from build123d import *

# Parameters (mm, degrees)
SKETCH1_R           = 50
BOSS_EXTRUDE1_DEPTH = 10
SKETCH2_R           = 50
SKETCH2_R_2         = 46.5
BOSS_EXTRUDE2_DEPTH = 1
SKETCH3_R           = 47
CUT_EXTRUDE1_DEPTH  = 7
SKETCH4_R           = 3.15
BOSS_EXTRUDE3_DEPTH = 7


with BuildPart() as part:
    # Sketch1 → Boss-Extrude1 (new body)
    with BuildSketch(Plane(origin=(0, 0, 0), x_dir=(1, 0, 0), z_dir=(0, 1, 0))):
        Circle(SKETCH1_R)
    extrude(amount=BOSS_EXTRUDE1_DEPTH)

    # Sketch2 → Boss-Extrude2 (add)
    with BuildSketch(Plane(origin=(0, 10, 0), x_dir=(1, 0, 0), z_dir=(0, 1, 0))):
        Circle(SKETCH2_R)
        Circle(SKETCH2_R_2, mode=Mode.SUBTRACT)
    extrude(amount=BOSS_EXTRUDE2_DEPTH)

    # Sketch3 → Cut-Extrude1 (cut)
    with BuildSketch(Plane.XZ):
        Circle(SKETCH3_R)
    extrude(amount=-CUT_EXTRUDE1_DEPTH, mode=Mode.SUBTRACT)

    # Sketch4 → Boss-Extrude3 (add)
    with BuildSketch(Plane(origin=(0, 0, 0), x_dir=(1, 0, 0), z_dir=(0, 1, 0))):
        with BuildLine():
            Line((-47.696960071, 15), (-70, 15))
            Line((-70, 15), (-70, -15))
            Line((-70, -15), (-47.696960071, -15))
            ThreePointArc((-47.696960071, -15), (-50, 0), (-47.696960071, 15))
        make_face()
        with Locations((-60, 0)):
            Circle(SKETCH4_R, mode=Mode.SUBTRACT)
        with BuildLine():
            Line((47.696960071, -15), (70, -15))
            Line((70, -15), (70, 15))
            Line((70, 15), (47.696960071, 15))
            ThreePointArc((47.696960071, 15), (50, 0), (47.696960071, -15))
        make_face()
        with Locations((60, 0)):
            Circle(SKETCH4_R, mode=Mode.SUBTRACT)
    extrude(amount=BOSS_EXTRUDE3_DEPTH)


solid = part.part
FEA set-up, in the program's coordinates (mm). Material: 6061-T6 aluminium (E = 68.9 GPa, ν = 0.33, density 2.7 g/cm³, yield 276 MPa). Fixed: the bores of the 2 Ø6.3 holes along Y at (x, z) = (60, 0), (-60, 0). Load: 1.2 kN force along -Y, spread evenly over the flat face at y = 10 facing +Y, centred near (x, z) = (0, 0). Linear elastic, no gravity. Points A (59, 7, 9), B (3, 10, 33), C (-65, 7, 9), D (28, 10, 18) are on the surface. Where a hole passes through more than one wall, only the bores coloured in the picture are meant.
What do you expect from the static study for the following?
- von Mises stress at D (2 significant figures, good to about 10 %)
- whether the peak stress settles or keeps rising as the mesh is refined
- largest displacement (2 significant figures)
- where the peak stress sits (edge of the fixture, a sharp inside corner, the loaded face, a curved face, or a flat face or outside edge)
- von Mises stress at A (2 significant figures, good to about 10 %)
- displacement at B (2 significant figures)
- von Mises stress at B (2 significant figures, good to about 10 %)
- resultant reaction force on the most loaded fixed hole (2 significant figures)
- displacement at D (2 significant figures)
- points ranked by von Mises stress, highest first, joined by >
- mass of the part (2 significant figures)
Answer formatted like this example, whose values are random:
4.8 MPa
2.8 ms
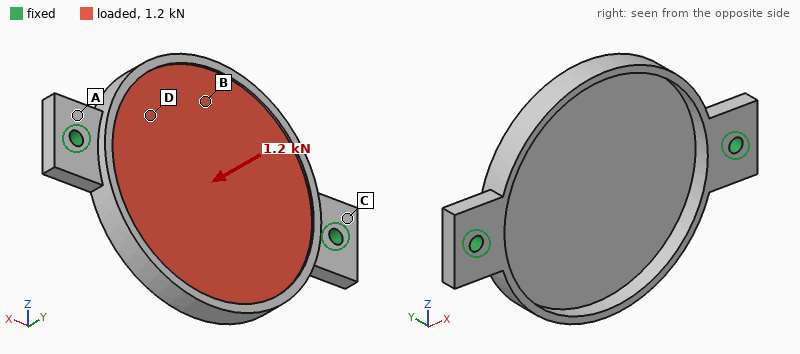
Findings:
17 MPa
keeps rising
0.18 mm
edge of the fixture
9.6 MPa
0.15 mm
24 MPa
1.4 kN
0.095 mm
B > D > A > C
110 g
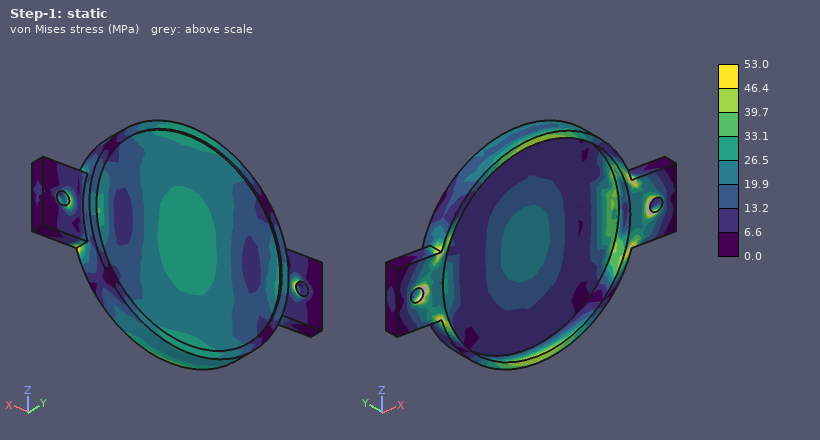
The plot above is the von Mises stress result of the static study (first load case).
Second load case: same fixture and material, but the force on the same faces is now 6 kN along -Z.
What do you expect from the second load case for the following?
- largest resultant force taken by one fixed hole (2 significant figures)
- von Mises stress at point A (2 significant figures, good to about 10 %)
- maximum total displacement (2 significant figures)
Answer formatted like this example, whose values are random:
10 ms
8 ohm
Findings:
3.0 kN
38 MPa
0.32 mm
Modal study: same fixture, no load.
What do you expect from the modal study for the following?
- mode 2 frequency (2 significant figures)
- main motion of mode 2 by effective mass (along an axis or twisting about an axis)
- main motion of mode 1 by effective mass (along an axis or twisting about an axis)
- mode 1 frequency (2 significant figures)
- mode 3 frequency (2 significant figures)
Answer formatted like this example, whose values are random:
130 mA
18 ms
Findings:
1700 Hz
along Y
twisting about X
1500 Hz
3200 Hz
